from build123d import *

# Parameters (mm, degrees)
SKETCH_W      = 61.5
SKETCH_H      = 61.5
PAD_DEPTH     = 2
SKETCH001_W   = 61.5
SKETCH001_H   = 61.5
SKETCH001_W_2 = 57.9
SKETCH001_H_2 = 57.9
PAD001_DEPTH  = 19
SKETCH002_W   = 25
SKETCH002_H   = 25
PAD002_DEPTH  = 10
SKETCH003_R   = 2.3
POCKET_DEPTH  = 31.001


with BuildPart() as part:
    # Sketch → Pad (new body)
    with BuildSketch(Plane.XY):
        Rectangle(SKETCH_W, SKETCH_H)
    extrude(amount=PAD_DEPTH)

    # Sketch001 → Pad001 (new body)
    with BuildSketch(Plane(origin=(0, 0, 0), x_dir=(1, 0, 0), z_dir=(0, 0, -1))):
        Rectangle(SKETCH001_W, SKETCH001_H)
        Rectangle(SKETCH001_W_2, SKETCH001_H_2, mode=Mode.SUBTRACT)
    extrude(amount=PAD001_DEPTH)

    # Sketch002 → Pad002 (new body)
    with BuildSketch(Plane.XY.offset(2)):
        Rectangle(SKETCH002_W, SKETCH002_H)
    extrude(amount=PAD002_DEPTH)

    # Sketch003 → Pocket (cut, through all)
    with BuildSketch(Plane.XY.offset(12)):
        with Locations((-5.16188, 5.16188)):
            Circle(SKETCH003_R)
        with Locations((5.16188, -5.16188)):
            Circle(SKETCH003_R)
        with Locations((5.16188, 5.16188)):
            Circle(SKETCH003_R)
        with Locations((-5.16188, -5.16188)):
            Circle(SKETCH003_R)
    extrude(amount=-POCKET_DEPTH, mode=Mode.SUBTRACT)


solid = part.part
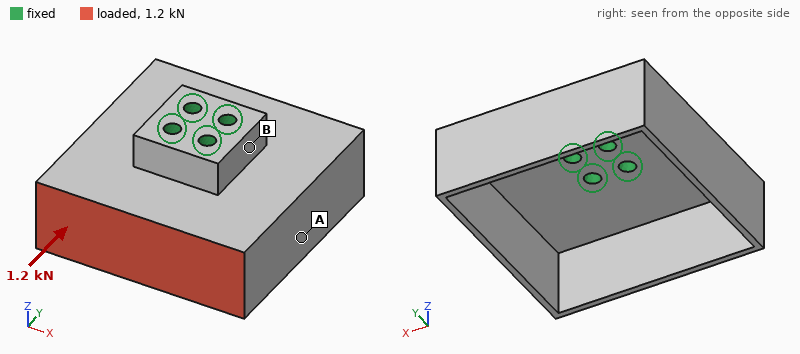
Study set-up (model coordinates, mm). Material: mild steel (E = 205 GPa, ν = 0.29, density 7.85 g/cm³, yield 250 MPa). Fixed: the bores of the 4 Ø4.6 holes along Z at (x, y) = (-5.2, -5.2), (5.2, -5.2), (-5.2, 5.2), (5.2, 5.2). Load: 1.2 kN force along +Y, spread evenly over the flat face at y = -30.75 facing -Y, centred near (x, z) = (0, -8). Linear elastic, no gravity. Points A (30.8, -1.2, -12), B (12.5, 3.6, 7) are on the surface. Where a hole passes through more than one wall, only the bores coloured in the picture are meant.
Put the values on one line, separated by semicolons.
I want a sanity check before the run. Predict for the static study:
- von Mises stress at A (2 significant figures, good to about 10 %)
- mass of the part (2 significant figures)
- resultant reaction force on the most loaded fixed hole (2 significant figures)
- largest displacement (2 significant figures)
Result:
24 MPa; 170 g; 530 N; 0.23 mm
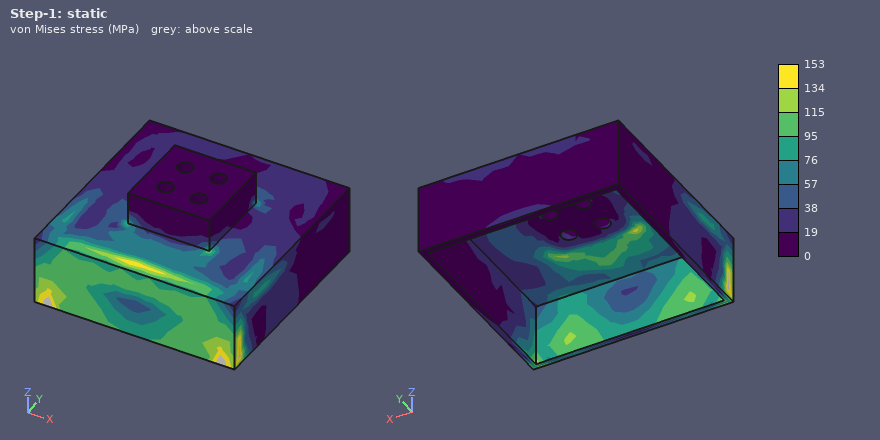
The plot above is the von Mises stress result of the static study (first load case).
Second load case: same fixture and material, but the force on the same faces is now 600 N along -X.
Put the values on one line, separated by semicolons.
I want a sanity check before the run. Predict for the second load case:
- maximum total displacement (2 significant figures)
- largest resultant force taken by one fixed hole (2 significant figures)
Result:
89 µm; 710 N
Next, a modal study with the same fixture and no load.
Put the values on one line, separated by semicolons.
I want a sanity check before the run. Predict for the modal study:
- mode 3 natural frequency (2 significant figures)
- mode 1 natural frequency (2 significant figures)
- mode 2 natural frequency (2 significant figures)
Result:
1800 Hz; 1600 Hz; 1800 Hz
